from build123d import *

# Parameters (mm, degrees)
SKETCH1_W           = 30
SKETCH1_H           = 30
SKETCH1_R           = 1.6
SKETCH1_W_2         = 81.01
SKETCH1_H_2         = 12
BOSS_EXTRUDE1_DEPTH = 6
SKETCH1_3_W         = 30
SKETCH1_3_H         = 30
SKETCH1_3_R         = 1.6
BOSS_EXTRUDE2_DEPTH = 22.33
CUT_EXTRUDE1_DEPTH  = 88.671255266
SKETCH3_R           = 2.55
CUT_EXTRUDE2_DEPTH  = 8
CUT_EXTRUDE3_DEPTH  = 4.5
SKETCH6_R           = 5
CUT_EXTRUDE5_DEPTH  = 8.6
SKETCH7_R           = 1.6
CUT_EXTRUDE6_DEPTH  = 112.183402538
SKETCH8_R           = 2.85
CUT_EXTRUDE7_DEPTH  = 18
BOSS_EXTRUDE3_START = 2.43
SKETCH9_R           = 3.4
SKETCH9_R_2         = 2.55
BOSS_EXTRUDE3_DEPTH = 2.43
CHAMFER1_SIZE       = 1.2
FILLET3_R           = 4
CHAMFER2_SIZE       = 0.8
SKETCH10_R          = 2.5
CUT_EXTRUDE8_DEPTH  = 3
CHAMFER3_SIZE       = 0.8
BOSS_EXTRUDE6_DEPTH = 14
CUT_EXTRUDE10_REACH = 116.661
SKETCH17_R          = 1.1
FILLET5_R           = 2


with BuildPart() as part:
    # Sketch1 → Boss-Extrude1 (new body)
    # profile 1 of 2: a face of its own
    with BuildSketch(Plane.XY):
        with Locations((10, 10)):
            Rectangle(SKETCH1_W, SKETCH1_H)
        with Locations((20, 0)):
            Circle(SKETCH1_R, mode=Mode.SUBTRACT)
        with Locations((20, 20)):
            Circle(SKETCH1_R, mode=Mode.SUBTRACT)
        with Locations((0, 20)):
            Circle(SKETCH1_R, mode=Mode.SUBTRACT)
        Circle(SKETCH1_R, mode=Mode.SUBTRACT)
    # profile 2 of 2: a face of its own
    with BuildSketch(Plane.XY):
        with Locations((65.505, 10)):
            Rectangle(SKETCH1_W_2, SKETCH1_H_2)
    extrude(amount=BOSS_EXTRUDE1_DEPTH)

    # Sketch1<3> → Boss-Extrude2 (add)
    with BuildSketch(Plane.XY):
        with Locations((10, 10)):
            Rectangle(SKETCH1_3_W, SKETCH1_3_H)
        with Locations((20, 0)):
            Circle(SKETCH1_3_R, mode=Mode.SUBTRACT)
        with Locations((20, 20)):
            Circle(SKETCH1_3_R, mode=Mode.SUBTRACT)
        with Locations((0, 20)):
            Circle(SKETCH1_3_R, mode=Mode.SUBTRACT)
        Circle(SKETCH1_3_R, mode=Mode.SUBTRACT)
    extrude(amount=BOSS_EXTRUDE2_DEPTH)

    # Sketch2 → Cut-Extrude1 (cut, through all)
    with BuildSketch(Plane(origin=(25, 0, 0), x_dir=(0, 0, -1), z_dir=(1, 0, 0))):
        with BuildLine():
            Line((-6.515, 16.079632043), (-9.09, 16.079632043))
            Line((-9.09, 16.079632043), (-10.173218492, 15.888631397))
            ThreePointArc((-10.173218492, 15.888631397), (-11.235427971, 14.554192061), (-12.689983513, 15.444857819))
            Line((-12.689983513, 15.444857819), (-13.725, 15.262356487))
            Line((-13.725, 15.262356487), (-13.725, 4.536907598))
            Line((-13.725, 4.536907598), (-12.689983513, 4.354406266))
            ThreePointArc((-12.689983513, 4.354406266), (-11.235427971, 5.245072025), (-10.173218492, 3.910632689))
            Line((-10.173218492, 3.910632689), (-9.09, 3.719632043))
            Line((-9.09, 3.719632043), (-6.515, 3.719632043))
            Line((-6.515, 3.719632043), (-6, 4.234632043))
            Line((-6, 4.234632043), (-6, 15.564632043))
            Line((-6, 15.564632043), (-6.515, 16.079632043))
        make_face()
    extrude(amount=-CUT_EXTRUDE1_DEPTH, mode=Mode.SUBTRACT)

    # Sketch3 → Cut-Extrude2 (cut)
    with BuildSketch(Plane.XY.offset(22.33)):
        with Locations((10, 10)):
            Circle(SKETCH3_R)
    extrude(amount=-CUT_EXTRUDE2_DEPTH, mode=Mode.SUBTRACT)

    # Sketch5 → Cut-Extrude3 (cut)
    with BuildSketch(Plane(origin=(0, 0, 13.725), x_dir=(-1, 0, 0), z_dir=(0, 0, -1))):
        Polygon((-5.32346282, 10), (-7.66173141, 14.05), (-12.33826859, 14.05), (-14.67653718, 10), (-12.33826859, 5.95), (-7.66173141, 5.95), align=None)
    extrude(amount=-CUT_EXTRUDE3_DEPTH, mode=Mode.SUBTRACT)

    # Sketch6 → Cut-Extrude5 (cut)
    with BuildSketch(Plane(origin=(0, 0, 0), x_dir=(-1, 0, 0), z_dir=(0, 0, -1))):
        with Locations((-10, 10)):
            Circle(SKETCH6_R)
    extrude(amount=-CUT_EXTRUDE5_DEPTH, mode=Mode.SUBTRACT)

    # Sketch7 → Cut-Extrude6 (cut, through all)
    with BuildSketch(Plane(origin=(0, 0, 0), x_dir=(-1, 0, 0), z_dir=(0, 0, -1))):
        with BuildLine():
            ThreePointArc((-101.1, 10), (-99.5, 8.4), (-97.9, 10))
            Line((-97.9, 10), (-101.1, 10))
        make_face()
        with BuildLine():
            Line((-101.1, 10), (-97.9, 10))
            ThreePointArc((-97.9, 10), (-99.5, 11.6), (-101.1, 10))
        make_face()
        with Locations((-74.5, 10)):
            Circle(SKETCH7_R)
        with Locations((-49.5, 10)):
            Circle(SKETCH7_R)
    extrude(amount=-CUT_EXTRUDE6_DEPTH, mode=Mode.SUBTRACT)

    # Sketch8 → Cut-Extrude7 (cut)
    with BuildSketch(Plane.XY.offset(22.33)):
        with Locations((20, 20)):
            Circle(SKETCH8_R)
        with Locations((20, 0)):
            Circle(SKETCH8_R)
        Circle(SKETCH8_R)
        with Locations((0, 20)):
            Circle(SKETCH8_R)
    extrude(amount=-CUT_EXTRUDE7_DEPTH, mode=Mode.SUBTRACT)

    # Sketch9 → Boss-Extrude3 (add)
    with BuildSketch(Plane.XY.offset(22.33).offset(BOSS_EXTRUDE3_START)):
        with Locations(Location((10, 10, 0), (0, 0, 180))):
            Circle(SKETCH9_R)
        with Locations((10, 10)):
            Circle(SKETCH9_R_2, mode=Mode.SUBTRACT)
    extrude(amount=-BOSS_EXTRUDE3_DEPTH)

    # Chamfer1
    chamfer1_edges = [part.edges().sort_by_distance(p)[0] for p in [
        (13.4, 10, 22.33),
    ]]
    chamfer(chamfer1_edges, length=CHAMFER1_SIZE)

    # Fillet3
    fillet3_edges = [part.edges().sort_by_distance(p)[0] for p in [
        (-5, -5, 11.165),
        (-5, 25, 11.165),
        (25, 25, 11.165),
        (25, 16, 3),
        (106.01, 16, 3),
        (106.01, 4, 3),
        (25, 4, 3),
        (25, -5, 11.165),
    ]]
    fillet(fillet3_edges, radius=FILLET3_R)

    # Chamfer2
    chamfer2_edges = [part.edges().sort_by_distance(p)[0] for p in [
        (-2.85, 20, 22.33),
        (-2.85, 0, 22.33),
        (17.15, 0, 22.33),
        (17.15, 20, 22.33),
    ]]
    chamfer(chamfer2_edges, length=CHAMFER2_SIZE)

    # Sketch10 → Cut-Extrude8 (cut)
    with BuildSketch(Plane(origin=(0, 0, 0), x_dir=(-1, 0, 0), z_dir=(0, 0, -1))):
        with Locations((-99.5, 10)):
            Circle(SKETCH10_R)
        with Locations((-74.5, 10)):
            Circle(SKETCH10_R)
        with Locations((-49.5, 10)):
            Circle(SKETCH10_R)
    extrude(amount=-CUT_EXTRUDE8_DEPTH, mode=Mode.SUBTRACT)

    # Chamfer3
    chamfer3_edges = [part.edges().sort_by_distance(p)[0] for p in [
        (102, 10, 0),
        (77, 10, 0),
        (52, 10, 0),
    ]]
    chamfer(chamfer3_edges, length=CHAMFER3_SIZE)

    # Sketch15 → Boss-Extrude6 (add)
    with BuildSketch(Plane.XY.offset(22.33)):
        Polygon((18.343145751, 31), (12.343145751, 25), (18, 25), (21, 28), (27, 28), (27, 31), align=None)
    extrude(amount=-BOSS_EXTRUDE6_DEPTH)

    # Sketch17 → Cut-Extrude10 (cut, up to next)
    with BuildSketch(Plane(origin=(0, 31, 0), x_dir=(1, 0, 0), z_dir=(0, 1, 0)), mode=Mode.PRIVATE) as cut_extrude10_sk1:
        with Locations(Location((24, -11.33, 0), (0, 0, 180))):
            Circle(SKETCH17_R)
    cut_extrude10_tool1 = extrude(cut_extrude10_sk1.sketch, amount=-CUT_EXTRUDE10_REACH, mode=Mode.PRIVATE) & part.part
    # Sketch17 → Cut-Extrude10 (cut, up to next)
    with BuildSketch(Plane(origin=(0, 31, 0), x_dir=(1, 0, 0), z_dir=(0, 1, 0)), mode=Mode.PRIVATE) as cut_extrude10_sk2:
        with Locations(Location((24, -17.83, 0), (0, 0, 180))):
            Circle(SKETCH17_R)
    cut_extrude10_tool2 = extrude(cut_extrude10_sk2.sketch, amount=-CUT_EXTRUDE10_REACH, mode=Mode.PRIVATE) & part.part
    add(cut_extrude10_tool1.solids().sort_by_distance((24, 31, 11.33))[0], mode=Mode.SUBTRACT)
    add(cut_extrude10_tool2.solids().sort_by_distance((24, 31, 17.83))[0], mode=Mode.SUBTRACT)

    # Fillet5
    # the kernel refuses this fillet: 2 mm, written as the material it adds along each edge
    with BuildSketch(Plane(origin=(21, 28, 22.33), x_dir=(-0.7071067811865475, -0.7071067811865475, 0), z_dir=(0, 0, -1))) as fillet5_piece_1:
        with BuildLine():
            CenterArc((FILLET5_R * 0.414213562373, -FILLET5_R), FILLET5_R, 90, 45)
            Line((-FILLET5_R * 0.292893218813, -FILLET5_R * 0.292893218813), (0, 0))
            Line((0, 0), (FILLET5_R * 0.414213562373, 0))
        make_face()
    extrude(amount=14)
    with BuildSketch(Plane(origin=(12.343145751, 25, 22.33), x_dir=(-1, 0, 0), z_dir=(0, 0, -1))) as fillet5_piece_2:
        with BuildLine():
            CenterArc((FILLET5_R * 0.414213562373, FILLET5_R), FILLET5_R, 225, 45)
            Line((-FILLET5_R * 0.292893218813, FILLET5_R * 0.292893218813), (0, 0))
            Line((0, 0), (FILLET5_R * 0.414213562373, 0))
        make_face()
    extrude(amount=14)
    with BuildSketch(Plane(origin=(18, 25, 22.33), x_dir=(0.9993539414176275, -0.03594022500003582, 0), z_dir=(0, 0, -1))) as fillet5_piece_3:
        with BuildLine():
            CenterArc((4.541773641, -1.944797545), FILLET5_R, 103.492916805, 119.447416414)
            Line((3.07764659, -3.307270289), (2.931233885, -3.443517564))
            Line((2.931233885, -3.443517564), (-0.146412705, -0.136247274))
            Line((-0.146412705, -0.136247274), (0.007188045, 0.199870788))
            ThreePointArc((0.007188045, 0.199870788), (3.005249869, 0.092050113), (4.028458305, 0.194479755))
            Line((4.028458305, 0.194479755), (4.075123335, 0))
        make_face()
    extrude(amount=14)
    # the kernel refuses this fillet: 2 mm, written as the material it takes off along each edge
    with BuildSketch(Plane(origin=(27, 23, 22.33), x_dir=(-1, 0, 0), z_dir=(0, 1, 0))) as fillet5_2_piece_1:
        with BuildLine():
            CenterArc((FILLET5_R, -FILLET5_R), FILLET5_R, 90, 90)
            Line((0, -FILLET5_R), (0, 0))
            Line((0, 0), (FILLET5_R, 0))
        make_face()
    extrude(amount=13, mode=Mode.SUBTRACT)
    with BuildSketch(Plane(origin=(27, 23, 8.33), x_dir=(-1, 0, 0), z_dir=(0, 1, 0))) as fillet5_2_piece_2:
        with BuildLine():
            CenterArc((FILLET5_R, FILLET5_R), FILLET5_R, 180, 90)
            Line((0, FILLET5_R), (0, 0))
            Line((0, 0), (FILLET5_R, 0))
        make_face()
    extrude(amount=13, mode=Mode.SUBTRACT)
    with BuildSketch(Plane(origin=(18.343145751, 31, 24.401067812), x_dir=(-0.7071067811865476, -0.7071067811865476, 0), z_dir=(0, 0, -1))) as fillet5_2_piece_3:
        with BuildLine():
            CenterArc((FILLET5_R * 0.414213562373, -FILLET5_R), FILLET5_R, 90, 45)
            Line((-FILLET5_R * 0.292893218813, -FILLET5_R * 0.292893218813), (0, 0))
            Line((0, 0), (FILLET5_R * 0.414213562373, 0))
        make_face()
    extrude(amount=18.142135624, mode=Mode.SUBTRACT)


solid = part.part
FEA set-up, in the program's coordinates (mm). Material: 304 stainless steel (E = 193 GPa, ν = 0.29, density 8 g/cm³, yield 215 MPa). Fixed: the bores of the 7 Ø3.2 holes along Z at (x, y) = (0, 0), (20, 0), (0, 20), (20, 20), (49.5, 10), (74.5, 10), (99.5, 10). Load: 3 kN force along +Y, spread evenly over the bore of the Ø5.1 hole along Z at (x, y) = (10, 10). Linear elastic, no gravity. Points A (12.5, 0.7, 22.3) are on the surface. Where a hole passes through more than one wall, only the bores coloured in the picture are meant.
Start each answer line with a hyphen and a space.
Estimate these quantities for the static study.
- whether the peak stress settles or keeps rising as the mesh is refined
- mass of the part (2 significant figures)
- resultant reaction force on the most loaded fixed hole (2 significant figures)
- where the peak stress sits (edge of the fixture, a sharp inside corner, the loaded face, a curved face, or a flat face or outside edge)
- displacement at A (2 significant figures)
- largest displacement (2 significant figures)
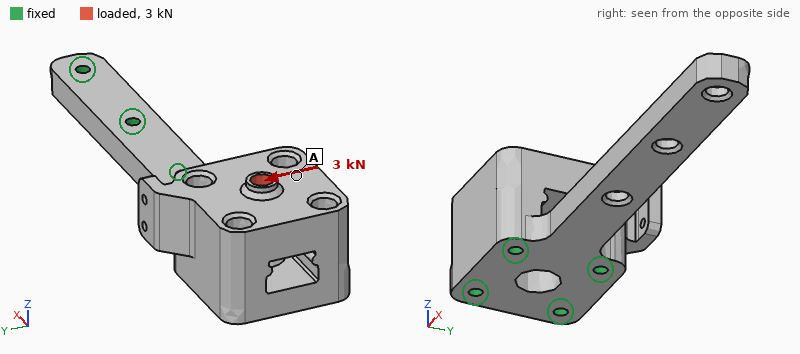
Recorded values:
- keeps rising
- 170 g
- 1.4 kN
- edge of the fixture
- 7.8 µm
- 11 µm
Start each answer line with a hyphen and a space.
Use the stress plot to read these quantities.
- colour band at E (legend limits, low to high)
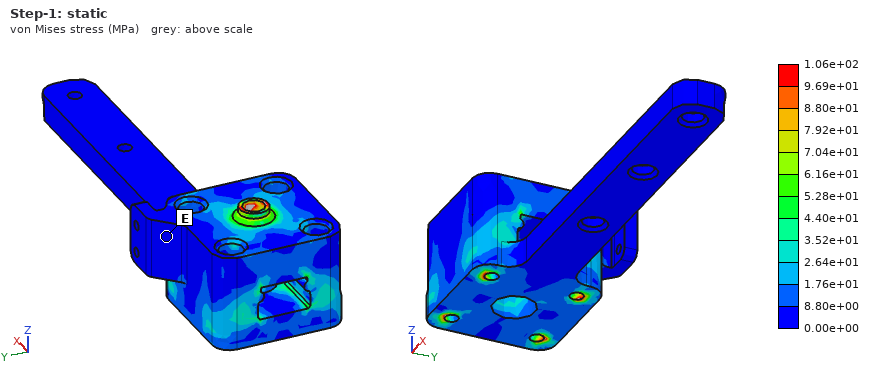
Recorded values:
- 0.00e+00 to 8.80e+00 MPa
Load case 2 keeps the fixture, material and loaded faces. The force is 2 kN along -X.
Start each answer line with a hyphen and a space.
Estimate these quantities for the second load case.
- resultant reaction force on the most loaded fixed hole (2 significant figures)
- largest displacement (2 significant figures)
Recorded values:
- 1.0 kN
- 6.1 µm
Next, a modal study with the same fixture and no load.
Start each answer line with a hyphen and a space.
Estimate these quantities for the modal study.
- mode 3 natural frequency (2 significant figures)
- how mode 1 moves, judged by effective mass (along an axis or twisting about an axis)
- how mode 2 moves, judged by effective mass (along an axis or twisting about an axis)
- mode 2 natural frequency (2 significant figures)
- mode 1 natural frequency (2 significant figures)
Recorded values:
- 22 kHz
- along Y
- along X
- 17 kHz
- 13 kHz
